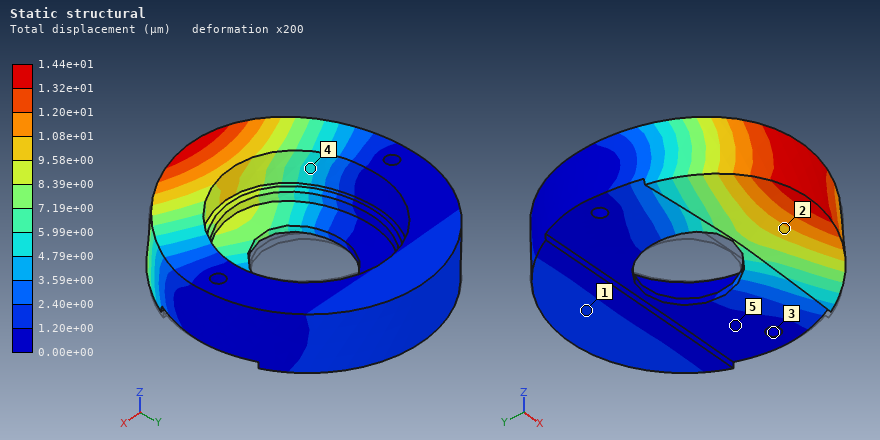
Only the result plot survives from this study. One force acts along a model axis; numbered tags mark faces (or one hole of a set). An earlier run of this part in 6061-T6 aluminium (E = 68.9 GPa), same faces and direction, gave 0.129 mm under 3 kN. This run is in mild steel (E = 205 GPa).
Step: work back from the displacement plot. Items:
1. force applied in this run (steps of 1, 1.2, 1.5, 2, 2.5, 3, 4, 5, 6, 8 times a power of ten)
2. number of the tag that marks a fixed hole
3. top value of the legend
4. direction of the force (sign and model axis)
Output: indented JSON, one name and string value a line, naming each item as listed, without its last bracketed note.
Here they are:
{
  "force applied in this run": "1 kN",
  "number of the tag that marks a fixed hole": "3",
  "top value of the legend": "1.44e+01 µm",
  "direction of the force": "+Z"
}
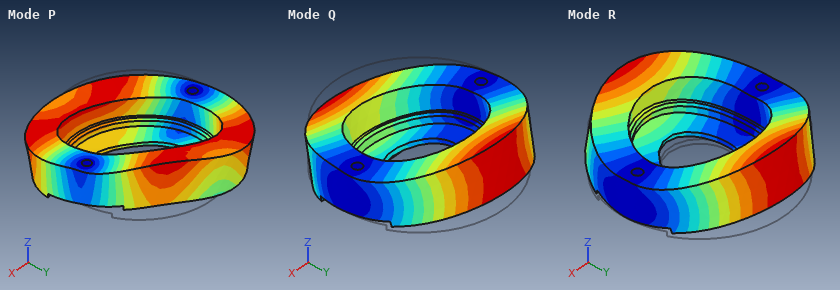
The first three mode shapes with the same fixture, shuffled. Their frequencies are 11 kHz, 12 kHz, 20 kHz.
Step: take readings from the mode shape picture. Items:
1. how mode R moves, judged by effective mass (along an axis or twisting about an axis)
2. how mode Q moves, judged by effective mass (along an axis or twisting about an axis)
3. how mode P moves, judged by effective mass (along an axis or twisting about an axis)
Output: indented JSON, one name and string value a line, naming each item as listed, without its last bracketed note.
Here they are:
{
  "how mode R moves, judged by effective mass": "along Z",
  "how mode Q moves, judged by effective mass": "twisting about X",
  "how mode P moves, judged by effective mass": "twisting about Z"
}
